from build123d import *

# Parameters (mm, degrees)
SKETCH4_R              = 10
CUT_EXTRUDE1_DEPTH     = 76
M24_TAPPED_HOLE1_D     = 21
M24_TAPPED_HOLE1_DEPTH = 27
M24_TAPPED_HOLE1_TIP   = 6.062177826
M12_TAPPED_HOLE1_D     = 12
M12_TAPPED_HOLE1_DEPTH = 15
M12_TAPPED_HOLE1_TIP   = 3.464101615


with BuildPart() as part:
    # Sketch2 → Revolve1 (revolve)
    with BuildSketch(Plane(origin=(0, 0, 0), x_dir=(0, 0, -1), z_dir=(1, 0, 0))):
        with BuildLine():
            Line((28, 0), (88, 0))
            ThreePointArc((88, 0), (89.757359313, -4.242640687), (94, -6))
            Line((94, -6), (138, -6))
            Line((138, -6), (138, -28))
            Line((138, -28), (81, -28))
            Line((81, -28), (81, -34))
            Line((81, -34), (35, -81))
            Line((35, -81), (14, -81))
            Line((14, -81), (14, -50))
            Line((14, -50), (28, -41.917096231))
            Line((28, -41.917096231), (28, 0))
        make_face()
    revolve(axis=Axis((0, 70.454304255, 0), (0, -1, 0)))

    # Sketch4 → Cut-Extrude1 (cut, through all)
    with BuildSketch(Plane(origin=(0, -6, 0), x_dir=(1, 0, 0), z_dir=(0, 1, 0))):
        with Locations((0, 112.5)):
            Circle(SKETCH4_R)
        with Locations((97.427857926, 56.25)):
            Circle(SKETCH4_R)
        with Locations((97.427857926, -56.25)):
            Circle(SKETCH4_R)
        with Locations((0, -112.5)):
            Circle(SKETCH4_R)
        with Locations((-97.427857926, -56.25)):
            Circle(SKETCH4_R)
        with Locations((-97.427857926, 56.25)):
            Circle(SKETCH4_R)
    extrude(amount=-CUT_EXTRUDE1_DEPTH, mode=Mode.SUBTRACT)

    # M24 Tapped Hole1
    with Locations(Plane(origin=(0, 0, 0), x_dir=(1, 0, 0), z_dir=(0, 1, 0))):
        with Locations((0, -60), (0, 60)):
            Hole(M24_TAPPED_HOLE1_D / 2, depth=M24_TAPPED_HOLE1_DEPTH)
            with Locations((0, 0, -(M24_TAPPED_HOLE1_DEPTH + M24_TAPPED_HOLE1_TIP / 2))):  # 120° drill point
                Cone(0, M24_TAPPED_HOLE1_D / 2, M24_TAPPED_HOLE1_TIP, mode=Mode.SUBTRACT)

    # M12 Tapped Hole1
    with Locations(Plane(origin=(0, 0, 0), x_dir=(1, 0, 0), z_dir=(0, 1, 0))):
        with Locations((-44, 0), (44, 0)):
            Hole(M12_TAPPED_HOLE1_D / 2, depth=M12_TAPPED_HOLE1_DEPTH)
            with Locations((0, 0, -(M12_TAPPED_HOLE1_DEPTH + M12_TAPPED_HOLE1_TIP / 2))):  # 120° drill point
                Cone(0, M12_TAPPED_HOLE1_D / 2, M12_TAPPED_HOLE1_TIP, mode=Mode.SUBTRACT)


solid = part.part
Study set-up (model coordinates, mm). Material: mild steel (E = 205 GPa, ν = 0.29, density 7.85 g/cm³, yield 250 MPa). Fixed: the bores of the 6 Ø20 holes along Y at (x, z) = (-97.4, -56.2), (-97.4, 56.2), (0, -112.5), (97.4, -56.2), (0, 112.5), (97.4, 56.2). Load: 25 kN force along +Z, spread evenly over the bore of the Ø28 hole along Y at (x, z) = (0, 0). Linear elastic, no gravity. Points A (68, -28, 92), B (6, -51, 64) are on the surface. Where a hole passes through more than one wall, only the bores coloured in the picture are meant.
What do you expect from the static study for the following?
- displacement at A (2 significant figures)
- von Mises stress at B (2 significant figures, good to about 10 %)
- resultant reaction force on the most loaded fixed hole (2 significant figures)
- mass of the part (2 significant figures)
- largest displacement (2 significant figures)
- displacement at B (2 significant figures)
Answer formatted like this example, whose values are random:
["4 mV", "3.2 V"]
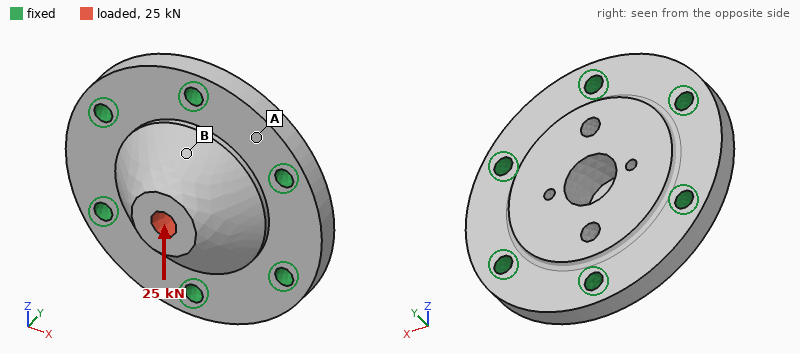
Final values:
["0.98 µm", "6.2 MPa", "7.2 kN", "15 kg", "5.6 µm", "3.1 µm"]
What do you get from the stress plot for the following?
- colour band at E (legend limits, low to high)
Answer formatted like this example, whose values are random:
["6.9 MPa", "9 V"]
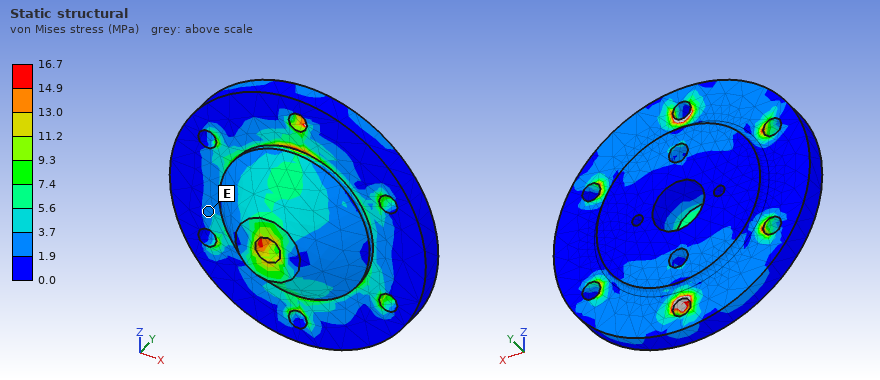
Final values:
["1.9 to 3.7 MPa"]
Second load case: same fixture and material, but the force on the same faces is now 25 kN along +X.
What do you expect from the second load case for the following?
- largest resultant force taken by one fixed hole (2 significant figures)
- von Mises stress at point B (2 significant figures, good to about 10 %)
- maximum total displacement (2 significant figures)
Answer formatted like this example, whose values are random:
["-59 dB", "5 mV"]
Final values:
["6.4 kN", "1.7 MPa", "5.5 µm"]
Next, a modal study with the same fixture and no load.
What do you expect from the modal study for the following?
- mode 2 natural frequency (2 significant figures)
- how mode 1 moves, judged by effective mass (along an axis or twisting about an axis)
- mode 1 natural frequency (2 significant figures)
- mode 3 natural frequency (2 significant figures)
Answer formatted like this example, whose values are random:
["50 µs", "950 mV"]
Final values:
["6200 Hz", "along Y", "4300 Hz", "6200 Hz"]
